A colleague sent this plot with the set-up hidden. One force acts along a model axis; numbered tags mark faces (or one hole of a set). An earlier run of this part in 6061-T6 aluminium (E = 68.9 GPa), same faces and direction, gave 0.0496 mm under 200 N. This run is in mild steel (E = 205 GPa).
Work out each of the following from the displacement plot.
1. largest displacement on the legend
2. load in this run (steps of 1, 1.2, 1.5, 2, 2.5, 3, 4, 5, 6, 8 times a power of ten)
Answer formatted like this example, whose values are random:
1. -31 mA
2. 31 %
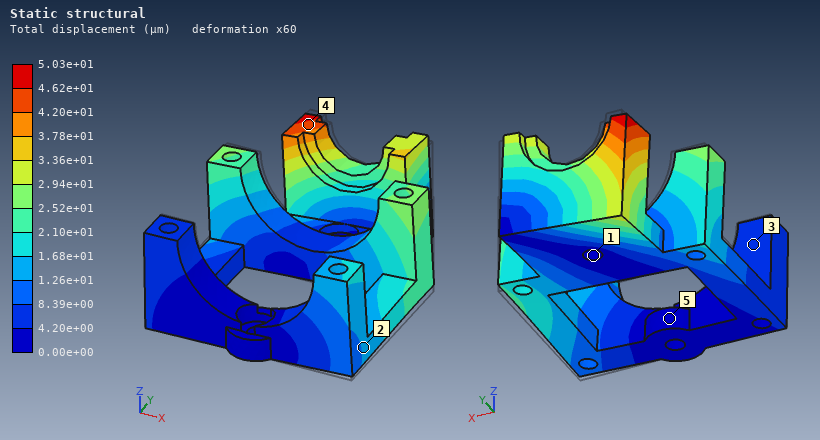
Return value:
1. 5.03e+01 µm
2. 600 N
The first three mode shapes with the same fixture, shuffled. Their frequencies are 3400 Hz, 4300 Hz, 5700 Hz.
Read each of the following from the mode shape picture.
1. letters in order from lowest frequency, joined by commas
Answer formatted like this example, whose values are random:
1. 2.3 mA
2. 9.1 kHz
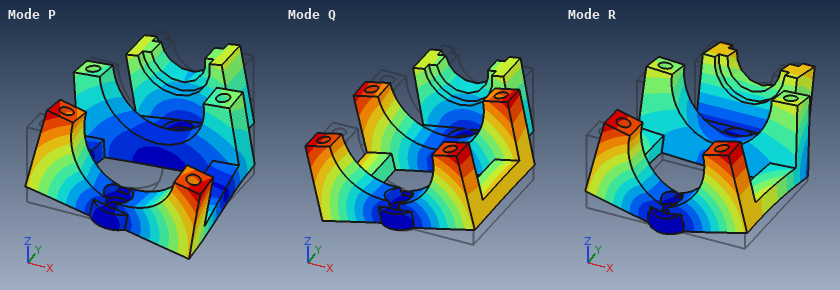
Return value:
1. Q, R, P
